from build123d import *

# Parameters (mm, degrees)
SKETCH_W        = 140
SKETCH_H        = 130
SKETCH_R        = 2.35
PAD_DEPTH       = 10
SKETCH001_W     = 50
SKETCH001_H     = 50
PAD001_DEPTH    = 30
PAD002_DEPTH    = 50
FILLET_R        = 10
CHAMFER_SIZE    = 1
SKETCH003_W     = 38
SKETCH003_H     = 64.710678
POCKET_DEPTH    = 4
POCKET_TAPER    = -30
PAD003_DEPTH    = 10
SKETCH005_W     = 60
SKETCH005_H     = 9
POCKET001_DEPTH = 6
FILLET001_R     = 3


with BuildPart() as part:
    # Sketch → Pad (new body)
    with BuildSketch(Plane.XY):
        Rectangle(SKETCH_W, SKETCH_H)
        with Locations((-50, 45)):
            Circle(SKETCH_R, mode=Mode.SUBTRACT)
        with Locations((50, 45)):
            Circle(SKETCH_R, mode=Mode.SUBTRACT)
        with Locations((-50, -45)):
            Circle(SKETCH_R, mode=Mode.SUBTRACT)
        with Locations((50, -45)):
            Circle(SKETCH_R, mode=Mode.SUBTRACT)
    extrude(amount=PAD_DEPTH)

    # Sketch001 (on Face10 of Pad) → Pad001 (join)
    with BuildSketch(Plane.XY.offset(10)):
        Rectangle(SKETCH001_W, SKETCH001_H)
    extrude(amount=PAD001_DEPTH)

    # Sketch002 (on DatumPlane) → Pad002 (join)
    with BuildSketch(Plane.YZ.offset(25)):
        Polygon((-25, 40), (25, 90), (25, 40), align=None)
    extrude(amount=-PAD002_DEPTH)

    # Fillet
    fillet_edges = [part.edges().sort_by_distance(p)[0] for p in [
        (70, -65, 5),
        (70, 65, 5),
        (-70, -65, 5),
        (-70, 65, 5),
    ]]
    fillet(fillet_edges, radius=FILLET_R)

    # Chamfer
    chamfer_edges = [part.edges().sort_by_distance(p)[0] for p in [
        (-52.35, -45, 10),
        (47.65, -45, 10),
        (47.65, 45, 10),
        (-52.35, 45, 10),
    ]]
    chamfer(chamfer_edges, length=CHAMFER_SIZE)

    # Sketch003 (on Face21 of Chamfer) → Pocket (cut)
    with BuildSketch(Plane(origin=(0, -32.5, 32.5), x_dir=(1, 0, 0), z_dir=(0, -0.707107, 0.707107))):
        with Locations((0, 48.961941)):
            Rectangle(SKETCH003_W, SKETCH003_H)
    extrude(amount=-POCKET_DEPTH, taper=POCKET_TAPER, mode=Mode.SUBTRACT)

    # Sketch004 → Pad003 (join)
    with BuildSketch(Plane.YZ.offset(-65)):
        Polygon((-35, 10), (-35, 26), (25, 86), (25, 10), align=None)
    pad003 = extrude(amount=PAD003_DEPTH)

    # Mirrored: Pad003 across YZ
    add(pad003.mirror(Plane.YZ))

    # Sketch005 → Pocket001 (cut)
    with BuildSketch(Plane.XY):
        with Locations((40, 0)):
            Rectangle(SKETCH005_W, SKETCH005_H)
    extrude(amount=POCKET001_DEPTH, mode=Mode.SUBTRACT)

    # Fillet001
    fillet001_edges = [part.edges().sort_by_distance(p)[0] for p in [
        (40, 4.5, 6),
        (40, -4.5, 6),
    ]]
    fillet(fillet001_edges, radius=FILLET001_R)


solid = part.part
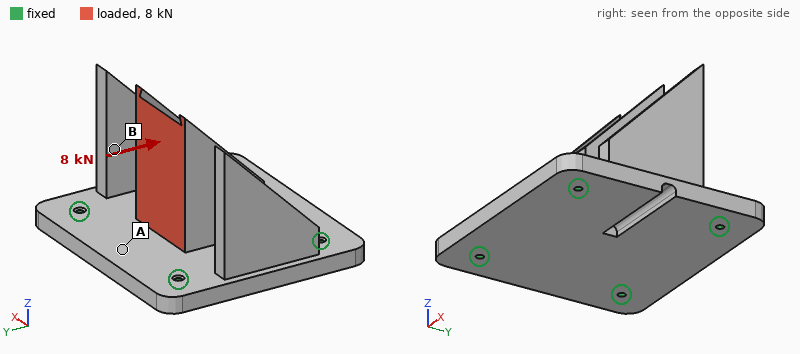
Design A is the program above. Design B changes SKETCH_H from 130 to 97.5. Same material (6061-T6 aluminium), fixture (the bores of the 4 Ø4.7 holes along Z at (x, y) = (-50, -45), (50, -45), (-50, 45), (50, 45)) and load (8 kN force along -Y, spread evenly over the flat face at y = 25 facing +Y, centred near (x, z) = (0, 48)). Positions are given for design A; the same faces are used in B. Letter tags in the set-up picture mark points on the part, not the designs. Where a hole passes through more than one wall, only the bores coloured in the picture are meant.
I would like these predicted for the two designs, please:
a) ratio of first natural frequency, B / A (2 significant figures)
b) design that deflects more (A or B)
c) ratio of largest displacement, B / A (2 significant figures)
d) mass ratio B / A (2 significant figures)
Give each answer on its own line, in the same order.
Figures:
0.98
B
1.2
0.87
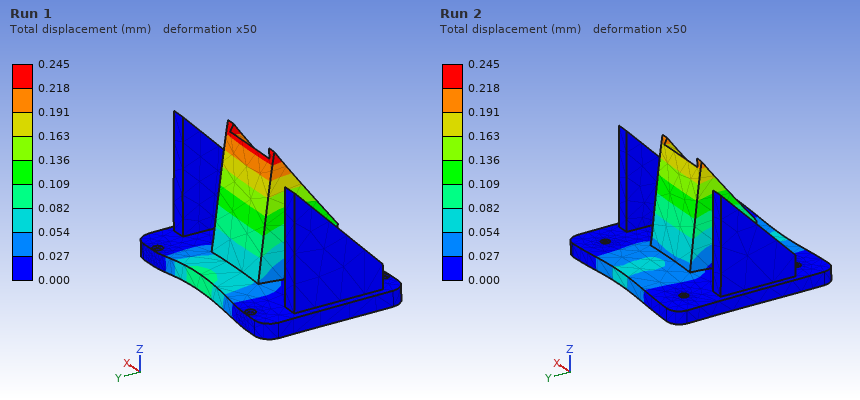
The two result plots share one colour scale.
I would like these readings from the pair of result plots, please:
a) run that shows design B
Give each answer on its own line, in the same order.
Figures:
Run 1
